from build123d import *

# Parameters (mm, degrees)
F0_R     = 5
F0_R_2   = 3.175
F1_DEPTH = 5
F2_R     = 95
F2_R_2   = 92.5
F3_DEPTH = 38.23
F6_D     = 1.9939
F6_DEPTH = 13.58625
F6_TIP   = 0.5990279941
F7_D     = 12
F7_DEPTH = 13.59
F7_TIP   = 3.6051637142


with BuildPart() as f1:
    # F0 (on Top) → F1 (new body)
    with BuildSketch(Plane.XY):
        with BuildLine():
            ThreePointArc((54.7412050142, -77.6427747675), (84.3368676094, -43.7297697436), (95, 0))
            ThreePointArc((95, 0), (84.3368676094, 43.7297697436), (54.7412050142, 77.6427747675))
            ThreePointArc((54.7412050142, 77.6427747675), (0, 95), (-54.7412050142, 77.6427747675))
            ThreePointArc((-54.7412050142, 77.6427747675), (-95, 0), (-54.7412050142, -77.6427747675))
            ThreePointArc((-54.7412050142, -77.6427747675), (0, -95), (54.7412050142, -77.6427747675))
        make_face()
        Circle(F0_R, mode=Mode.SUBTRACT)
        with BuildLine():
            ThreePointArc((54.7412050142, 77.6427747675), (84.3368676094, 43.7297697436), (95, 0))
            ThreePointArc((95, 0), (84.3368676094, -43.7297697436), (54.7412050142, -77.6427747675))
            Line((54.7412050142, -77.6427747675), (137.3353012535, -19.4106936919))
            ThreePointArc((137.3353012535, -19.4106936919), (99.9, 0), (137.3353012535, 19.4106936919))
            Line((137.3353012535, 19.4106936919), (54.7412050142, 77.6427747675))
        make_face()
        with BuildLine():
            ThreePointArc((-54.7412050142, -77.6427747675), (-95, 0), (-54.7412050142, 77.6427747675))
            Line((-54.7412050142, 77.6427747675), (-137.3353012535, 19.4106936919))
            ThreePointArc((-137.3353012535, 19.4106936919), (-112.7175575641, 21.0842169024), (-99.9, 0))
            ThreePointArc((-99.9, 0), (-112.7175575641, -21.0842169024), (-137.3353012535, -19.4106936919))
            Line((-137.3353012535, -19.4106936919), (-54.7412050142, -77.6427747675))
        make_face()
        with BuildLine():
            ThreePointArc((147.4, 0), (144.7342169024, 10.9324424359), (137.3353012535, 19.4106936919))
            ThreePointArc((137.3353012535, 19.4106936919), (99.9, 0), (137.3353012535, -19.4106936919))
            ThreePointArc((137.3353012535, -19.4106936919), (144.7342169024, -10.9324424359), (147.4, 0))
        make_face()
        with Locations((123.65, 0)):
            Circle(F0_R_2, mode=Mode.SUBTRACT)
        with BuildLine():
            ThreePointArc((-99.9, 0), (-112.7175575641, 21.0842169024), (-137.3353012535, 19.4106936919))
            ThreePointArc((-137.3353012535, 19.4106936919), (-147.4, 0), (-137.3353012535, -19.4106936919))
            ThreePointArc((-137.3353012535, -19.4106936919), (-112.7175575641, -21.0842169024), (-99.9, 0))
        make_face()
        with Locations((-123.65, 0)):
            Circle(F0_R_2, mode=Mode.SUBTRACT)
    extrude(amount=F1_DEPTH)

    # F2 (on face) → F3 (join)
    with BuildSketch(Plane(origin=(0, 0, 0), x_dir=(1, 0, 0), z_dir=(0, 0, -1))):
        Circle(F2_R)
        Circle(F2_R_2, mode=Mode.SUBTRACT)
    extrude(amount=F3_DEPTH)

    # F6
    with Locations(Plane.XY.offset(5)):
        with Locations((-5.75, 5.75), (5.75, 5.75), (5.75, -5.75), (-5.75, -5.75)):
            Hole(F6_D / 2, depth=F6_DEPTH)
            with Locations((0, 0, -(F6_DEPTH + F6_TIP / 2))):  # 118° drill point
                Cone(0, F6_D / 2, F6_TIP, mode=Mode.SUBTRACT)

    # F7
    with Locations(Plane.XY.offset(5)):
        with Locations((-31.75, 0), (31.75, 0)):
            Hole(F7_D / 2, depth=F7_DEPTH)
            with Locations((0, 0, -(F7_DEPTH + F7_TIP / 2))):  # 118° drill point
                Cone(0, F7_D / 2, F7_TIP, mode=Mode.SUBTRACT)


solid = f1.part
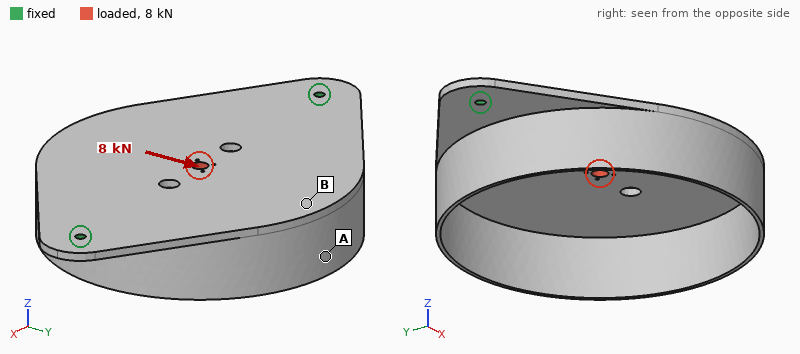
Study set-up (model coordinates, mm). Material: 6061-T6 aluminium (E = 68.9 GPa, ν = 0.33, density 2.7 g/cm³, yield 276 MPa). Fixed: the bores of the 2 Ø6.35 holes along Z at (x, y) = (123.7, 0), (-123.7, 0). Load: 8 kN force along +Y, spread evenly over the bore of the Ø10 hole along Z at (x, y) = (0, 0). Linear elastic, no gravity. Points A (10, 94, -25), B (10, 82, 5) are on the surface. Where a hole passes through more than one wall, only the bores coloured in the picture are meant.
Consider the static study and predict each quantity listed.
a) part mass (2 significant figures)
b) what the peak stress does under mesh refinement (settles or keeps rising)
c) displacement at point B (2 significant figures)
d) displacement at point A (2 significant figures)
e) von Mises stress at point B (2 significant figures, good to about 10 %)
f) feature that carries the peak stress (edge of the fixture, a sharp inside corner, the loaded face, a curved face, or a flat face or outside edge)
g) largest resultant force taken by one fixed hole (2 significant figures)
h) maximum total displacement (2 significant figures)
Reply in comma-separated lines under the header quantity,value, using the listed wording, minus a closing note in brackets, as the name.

quantity,value
part mass,640 g
what the peak stress does under mesh refinement,keeps rising
displacement at point B,47 µm
displacement at point A,19 µm
von Mises stress at point B,11 MPa
feature that carries the peak stress,edge of the fixture
largest resultant force taken by one fixed hole,4.0 kN
maximum total displacement,65 µm
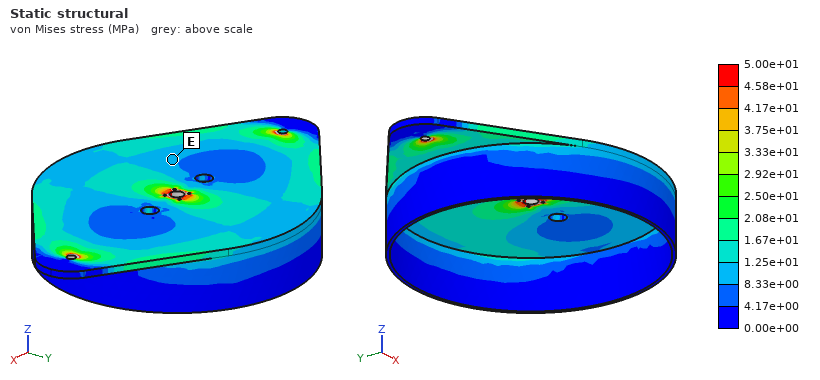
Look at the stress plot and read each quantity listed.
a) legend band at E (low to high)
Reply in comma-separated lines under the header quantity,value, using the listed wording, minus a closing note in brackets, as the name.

quantity,value
legend band at E,8.33e+00 to 1.25e+01 MPa
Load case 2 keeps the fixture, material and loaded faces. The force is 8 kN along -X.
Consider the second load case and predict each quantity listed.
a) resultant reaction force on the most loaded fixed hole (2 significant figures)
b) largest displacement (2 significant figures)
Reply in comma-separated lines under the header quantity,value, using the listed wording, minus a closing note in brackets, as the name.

quantity,value
resultant reaction force on the most loaded fixed hole,4.0 kN
largest displacement,35 µm
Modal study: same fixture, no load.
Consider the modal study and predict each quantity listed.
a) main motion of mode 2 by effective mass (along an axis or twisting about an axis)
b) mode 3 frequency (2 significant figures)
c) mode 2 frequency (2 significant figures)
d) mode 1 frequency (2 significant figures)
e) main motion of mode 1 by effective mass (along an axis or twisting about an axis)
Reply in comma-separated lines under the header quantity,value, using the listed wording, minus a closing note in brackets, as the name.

quantity,value
main motion of mode 2 by effective mass,along Z
mode 3 frequency,860 Hz
mode 2 frequency,330 Hz
mode 1 frequency,240 Hz
main motion of mode 1 by effective mass,twisting about X
